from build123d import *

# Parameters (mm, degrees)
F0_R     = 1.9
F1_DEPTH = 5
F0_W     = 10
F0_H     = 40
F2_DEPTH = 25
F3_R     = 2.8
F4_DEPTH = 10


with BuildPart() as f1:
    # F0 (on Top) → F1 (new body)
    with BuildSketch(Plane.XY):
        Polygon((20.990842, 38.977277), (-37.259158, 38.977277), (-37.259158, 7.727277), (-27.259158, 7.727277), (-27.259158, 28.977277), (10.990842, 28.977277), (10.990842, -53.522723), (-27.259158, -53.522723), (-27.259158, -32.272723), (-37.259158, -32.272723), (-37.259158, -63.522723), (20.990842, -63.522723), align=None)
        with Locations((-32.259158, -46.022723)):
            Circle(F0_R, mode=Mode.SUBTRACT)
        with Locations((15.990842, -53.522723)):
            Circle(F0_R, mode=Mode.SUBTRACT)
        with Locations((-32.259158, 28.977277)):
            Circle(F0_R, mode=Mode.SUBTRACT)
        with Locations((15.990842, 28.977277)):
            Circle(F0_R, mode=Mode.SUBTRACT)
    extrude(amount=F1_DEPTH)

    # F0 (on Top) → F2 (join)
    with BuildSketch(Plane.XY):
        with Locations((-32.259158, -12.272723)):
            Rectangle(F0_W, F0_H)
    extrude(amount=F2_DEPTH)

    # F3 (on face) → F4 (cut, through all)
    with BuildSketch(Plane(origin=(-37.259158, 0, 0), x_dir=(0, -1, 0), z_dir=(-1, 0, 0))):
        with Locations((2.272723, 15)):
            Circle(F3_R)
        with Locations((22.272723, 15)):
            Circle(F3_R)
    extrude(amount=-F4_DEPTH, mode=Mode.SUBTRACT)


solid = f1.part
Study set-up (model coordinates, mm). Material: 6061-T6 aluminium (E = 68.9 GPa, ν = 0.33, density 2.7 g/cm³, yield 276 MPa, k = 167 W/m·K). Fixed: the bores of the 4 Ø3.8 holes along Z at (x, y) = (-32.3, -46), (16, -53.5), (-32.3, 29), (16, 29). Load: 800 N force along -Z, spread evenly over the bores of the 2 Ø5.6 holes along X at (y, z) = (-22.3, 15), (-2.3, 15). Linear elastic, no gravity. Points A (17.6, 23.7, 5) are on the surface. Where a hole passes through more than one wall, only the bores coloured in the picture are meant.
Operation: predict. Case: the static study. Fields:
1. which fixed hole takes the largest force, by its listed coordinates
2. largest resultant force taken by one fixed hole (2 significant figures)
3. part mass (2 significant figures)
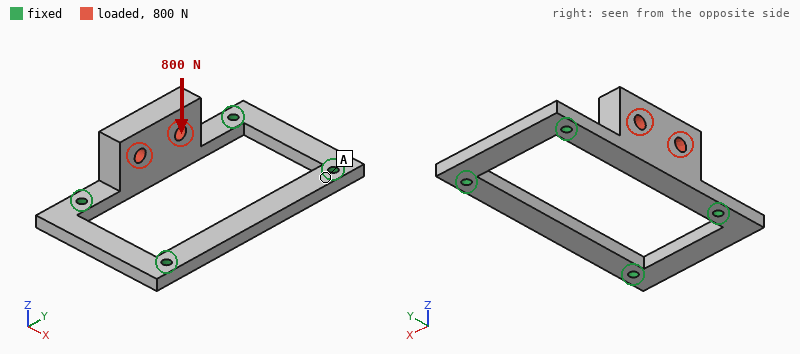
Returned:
(-32.3, -46)
510 N
58 g
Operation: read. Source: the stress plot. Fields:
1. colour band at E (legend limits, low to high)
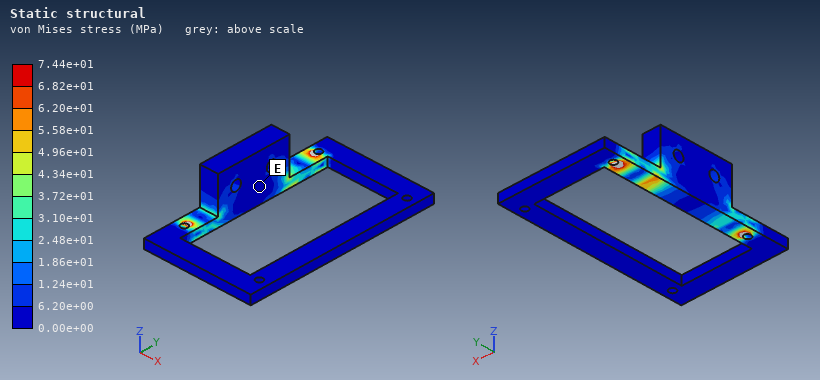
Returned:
0.00e+00 to 6.20e+00 MPa
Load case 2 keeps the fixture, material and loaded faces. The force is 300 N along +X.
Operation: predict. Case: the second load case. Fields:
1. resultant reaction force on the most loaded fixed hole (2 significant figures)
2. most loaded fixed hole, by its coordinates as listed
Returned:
200 N
(-32.3, -46)
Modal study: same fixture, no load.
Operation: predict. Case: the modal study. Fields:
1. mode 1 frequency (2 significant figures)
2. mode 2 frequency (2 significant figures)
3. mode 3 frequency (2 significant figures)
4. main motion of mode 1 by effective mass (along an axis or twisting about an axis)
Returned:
2200 Hz
3900 Hz
4000 Hz
along X
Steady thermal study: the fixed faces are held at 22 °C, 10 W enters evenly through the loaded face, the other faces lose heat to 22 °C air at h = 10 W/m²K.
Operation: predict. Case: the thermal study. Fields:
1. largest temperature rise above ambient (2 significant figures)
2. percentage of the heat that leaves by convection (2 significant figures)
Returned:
14 K
4.4 %
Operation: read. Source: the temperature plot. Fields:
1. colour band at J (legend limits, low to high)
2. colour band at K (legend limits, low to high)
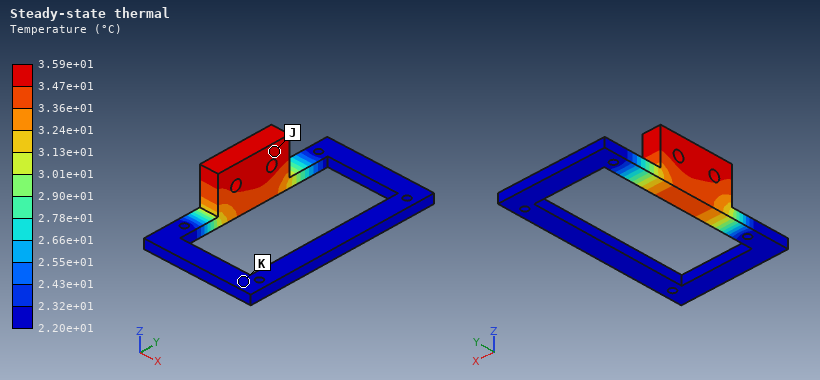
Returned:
3.47e+01 to 3.59e+01 °C
2.20e+01 to 2.32e+01 °C
